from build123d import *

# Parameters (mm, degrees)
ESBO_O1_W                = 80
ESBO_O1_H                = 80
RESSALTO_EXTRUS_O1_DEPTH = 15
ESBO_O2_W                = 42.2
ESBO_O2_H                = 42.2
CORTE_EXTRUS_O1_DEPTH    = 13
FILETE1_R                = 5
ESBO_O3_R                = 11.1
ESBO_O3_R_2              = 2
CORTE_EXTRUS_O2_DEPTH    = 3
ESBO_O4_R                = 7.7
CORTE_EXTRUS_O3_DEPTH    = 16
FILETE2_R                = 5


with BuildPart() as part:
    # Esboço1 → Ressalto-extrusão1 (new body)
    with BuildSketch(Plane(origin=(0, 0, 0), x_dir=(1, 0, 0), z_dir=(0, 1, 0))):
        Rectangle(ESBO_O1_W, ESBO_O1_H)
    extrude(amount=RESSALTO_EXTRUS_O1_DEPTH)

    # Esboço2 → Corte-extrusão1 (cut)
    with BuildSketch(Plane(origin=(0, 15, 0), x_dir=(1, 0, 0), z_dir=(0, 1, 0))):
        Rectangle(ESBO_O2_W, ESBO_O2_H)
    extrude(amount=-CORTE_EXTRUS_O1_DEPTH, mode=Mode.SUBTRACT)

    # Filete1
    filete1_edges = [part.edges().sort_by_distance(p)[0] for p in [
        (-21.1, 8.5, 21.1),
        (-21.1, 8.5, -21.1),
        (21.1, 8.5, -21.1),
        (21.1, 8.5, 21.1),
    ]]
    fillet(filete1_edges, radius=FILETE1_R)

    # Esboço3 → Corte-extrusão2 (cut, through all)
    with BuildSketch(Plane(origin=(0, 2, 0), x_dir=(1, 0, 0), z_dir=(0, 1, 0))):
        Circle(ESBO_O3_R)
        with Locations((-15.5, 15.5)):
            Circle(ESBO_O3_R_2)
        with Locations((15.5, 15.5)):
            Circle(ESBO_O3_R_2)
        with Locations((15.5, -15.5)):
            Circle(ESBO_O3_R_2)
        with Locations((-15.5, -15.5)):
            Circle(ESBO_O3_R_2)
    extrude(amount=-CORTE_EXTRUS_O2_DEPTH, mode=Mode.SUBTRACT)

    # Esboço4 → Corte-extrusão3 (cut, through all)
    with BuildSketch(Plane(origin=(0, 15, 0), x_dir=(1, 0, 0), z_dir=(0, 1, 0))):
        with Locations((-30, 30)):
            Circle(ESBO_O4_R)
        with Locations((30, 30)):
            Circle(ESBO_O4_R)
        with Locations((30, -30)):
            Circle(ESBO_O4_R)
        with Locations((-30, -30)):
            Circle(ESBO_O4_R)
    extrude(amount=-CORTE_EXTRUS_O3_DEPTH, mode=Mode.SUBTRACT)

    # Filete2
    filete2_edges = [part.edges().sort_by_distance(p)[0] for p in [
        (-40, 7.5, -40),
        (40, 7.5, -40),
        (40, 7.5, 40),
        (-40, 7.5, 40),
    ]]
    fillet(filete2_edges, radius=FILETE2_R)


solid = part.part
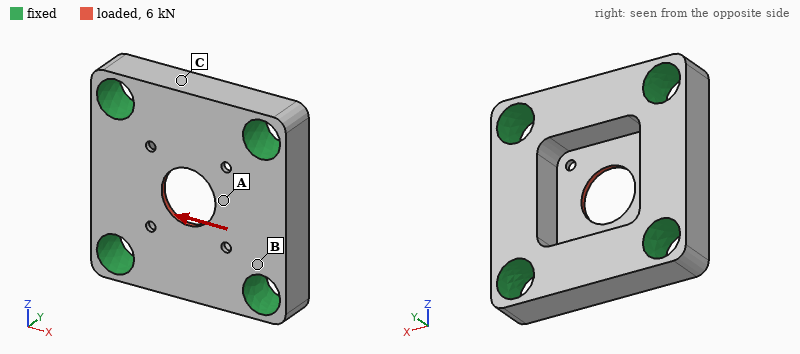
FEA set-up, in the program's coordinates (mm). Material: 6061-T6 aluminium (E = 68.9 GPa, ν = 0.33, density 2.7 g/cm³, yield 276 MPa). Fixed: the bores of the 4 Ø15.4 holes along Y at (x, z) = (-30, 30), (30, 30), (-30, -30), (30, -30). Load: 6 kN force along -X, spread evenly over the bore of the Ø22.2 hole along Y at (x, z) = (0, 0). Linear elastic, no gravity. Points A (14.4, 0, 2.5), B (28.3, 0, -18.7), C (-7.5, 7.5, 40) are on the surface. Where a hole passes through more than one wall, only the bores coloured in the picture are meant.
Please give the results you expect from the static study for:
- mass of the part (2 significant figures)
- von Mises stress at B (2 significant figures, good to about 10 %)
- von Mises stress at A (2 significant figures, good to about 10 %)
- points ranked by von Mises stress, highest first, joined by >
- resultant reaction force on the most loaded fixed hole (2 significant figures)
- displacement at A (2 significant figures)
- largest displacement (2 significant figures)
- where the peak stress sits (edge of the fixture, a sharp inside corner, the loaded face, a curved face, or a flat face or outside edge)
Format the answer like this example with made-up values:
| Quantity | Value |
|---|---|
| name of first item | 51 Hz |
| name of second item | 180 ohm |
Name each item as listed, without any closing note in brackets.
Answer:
| Quantity | Value |
|---|---|
| mass of the part | 160 g |
| von Mises stress at B | 18 MPa |
| von Mises stress at A | 38 MPa |
| points ranked by von Mises stress, highest first, joined by > | A > B > C |
| resultant reaction force on the most loaded fixed hole | 1.6 kN |
| displacement at A | 13 µm |
| largest displacement | 16 µm |
| where the peak stress sits | a sharp inside corner |
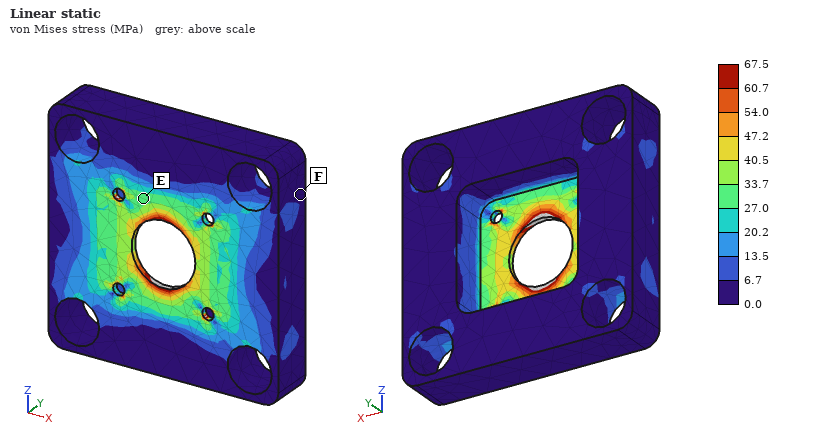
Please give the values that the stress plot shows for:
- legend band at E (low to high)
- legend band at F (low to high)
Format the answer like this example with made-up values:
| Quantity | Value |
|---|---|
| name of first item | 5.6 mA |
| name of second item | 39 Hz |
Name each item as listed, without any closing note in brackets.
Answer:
| Quantity | Value |
|---|---|
| legend band at E | 27.0 to 33.7 MPa |
| legend band at F | 0.0 to 6.7 MPa |
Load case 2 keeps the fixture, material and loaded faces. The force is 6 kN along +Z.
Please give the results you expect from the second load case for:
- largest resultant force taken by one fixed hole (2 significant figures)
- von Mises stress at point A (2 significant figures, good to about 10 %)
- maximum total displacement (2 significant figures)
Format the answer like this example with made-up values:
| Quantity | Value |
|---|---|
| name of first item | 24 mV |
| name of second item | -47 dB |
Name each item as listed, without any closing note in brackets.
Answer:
| Quantity | Value |
|---|---|
| largest resultant force taken by one fixed hole | 1.6 kN |
| von Mises stress at point A | 39 MPa |
| maximum total displacement | 16 µm |
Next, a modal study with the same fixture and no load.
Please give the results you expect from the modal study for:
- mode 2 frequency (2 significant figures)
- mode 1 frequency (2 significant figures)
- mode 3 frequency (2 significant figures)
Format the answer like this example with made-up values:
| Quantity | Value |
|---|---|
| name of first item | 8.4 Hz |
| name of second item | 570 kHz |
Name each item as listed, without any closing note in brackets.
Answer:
| Quantity | Value |
|---|---|
| mode 2 frequency | 16 kHz |
| mode 1 frequency | 13 kHz |
| mode 3 frequency | 17 kHz |
